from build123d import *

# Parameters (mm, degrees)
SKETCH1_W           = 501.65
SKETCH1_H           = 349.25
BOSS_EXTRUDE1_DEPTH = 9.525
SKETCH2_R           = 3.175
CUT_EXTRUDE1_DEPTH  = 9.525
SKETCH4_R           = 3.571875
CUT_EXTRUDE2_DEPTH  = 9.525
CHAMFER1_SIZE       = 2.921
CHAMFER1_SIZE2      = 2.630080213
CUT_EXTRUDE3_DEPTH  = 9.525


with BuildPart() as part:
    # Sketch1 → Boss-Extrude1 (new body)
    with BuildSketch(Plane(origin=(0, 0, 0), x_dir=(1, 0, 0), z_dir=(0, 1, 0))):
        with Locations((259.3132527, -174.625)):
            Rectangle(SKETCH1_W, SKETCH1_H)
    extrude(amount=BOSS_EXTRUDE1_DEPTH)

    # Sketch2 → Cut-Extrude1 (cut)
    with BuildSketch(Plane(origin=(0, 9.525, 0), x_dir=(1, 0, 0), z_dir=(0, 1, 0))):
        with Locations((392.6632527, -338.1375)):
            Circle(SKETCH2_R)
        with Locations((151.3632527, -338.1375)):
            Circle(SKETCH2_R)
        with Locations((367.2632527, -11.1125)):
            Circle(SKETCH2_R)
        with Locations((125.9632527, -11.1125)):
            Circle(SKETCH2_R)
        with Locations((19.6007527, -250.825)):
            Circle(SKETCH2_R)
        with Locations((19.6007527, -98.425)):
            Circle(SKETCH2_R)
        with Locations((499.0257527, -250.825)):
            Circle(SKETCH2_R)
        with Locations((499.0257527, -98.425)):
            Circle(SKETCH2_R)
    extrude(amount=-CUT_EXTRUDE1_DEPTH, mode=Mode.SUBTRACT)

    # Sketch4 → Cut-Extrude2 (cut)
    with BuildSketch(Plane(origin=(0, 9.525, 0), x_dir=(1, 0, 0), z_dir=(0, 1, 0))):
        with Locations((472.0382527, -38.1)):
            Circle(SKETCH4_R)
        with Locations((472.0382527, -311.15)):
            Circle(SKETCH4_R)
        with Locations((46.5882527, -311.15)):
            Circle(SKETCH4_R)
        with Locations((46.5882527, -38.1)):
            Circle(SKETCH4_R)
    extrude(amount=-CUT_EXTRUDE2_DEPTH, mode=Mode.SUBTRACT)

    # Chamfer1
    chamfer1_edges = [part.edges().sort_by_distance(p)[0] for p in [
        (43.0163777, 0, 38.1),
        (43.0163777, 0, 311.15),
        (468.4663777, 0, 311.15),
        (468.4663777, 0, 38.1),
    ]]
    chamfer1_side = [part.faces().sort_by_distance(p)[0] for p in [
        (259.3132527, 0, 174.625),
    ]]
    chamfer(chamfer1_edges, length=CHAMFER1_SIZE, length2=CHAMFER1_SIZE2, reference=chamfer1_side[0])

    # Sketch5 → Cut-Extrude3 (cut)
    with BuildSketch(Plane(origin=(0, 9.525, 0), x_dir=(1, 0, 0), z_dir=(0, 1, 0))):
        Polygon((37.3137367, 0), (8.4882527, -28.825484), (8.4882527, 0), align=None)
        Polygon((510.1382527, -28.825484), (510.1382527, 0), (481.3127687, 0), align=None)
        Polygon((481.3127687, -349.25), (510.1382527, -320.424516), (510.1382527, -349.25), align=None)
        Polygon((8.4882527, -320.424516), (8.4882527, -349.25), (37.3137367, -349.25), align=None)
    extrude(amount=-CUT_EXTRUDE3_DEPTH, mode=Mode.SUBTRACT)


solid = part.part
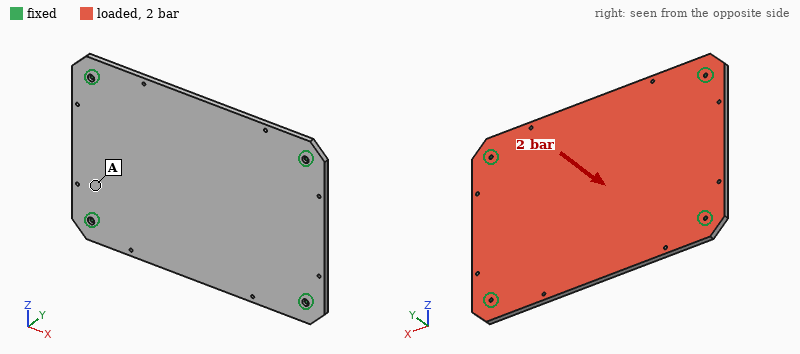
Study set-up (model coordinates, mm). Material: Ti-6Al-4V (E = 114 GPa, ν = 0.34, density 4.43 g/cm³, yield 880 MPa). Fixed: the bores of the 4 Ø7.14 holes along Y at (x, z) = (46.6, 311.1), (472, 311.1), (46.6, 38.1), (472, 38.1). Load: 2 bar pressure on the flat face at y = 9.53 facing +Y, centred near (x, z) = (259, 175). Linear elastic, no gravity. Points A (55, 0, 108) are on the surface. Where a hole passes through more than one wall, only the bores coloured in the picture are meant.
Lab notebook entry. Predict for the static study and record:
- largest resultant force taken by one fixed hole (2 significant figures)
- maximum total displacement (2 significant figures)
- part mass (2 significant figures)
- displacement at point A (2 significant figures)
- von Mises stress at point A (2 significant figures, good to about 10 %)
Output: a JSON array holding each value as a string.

["10 kN", "3.8 mm", "7.3 kg", "0.66 mm", "66 MPa"]
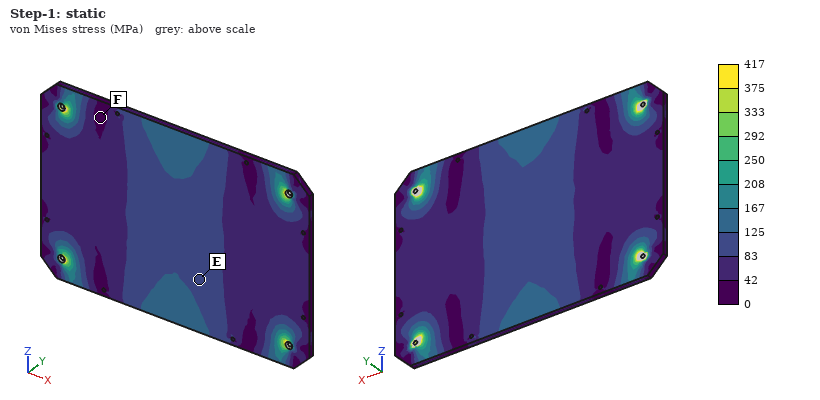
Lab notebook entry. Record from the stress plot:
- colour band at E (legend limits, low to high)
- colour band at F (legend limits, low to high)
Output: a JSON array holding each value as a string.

["83 to 125 MPa", "0 to 42 MPa"]
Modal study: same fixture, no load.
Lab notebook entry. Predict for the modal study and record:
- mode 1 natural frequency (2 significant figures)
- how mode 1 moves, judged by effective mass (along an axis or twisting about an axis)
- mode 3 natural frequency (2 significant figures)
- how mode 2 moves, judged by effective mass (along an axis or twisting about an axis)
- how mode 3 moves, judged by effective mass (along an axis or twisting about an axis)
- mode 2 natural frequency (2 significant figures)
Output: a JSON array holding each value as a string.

["200 Hz", "along Y", "510 Hz", "twisting about X", "twisting about Z", "320 Hz"]
